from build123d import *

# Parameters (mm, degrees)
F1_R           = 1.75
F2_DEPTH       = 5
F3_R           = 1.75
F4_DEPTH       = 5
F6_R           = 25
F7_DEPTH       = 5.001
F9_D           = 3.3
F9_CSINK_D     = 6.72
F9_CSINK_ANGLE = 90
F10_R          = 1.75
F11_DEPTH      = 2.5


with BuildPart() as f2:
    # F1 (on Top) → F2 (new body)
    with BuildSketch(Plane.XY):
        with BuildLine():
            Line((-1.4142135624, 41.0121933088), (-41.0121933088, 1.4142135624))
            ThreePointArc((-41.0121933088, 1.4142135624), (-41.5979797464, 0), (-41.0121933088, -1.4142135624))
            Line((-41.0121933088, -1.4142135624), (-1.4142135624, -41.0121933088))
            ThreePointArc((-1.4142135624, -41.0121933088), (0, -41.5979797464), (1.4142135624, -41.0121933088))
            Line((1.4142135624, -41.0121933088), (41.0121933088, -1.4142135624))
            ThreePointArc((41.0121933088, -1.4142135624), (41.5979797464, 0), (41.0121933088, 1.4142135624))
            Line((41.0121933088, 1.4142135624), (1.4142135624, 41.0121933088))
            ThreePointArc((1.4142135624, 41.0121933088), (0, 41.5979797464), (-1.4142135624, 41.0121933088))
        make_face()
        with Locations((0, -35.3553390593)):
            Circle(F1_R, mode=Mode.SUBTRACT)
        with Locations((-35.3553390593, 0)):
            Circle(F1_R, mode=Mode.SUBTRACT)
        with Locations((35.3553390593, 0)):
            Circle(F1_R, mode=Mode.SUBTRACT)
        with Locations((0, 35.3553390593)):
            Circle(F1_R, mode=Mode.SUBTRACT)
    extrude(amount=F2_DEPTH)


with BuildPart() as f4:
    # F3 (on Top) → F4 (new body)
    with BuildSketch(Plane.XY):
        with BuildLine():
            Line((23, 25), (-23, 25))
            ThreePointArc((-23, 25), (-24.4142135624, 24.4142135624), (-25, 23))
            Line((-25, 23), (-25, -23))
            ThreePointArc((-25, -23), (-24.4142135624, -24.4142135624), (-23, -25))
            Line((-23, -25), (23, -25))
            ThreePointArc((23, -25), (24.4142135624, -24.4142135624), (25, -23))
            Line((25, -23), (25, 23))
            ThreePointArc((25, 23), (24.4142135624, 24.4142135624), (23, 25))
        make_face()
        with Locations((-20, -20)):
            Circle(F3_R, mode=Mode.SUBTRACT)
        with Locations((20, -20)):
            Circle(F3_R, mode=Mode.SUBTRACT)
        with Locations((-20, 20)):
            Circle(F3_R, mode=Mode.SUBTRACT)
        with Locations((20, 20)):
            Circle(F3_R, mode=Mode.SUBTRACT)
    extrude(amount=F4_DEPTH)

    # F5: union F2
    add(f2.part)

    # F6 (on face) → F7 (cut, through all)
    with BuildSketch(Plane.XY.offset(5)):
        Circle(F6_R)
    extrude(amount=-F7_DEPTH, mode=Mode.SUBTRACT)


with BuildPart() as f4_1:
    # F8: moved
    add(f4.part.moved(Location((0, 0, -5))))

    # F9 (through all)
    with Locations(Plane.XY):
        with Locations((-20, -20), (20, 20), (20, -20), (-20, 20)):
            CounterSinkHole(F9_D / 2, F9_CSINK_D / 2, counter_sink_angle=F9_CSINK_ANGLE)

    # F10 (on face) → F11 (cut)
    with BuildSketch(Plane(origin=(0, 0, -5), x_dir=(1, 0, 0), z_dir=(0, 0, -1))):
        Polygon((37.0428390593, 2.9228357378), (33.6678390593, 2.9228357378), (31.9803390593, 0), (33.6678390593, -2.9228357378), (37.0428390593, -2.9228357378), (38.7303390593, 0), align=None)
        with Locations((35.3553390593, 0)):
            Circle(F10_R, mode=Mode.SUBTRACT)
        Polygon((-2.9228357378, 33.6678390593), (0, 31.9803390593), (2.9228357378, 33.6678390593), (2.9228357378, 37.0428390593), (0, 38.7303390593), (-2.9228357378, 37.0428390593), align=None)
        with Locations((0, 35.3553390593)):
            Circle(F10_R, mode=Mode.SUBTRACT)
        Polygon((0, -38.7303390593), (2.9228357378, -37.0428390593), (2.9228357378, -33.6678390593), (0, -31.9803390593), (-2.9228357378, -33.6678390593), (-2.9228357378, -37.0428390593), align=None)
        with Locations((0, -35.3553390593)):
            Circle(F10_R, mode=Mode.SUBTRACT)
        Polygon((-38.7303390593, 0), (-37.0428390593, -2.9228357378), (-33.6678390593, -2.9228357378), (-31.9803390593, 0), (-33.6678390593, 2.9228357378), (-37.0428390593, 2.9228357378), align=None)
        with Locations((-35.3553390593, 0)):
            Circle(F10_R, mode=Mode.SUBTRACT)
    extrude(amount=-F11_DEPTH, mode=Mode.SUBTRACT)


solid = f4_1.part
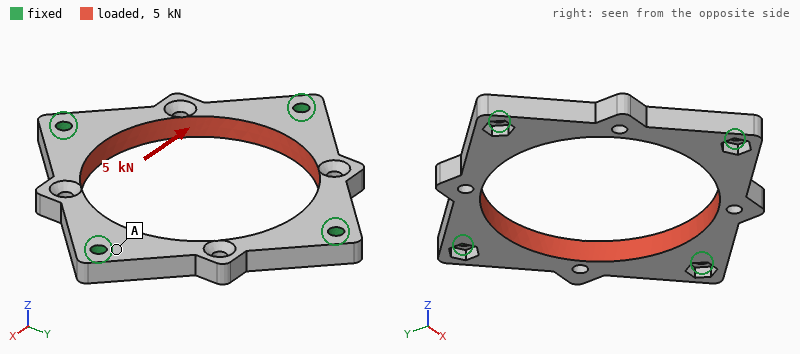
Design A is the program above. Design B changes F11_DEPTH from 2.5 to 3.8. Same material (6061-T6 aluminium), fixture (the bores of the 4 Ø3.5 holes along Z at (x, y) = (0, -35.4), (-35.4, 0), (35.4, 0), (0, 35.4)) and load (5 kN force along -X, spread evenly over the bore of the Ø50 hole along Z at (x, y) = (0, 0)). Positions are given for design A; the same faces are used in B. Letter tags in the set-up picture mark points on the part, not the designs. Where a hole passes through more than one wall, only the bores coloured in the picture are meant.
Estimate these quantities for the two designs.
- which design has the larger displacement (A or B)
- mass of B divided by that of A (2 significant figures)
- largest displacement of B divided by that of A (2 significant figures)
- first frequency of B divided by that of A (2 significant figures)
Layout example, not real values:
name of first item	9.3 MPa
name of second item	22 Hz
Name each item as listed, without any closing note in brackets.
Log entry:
which design has the larger displacement	B
mass of B divided by that of A	0.99
largest displacement of B divided by that of A	1.3
first frequency of B divided by that of A	0.79
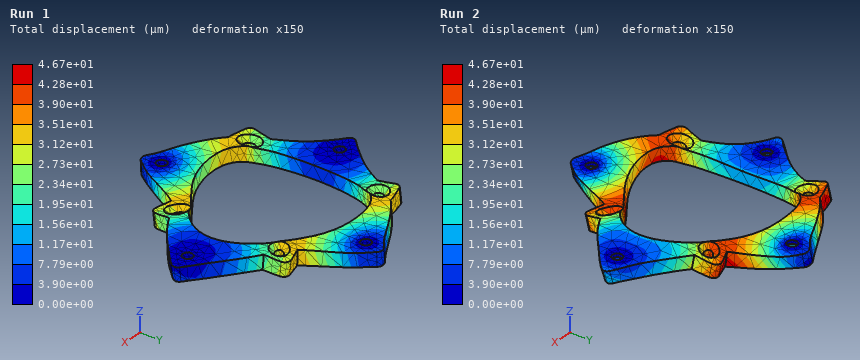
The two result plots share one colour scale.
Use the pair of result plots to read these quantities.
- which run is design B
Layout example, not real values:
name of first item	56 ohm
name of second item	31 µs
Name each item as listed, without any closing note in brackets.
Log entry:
which run is design B	Run 2
